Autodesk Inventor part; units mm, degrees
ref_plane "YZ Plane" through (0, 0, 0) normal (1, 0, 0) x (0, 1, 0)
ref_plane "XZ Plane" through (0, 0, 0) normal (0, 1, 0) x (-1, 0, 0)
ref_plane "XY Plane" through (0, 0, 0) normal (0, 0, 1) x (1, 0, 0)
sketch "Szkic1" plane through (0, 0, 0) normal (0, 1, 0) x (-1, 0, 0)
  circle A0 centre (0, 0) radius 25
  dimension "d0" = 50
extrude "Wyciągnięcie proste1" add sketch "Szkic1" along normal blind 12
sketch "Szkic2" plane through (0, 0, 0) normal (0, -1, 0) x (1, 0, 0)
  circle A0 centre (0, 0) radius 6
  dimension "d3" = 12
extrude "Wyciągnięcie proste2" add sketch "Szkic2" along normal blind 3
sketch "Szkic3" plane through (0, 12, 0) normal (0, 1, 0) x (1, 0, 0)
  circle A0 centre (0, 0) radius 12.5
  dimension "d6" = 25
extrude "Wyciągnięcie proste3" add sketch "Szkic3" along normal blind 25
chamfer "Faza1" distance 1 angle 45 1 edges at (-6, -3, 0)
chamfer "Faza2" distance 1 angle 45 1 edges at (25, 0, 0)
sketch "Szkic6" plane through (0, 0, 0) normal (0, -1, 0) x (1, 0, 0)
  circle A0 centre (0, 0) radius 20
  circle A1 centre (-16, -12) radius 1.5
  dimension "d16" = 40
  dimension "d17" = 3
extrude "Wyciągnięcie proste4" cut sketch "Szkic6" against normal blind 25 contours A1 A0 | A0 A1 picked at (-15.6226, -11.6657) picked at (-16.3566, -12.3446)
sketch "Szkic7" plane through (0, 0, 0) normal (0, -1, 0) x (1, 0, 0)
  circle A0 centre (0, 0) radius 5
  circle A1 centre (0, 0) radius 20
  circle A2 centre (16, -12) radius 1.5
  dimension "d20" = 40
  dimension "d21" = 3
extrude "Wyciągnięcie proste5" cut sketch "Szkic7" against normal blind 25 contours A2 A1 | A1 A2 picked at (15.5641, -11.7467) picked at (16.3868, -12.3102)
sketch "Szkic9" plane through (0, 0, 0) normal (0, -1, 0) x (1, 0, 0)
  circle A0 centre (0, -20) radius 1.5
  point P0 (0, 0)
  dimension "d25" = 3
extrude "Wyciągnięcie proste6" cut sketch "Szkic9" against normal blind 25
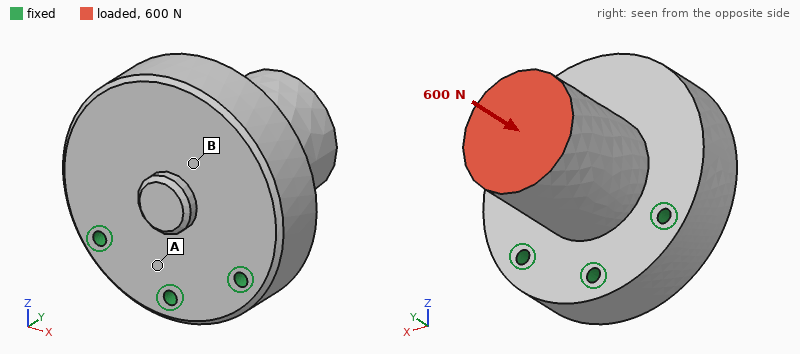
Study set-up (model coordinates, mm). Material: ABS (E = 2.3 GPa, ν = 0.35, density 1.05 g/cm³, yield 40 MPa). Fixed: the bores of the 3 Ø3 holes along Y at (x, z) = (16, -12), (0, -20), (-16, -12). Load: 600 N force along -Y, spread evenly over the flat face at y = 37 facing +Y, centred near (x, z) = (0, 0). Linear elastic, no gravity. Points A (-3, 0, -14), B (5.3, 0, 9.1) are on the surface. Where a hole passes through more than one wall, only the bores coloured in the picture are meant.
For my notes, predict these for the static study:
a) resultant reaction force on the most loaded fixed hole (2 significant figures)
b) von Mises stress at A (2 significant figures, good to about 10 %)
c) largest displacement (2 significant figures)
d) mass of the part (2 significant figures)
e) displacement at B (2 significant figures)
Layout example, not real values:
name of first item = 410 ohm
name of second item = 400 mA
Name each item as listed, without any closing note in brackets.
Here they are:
resultant reaction force on the most loaded fixed hole = 290 N
von Mises stress at A = 3.8 MPa
largest displacement = 0.22 mm
mass of the part = 38 g
displacement at B = 0.12 mm
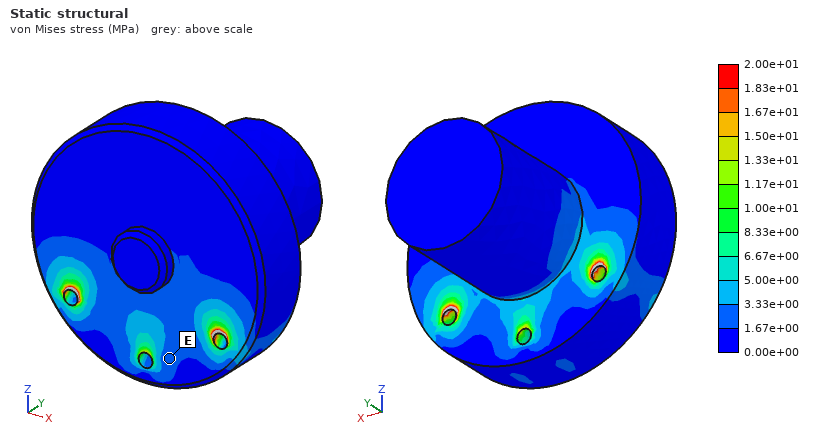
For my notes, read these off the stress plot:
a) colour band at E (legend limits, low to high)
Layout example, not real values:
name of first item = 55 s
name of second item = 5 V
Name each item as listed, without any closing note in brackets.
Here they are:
colour band at E = 1.67e+00 to 3.33e+00 MPa
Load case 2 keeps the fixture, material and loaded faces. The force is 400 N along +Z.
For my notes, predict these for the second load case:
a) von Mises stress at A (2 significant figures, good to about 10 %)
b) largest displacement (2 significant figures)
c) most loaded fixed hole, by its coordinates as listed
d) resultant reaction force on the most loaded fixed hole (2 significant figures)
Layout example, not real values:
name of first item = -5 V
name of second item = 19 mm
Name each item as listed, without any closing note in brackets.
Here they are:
von Mises stress at A = 6.6 MPa
largest displacement = 0.45 mm
most loaded fixed hole, by its coordinates as listed = (0, -20)
resultant reaction force on the most loaded fixed hole = 380 N
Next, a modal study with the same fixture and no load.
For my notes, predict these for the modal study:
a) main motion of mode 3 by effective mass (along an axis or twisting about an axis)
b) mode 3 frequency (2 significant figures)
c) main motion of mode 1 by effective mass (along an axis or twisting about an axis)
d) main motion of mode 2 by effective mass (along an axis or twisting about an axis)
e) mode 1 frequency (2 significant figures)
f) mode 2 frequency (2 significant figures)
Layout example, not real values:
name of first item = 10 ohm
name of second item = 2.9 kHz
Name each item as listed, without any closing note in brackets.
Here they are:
main motion of mode 3 by effective mass = along X
mode 3 frequency = 4400 Hz
main motion of mode 1 by effective mass = along Y
main motion of mode 2 by effective mass = along X
mode 1 frequency = 1500 Hz
mode 2 frequency = 3000 Hz
